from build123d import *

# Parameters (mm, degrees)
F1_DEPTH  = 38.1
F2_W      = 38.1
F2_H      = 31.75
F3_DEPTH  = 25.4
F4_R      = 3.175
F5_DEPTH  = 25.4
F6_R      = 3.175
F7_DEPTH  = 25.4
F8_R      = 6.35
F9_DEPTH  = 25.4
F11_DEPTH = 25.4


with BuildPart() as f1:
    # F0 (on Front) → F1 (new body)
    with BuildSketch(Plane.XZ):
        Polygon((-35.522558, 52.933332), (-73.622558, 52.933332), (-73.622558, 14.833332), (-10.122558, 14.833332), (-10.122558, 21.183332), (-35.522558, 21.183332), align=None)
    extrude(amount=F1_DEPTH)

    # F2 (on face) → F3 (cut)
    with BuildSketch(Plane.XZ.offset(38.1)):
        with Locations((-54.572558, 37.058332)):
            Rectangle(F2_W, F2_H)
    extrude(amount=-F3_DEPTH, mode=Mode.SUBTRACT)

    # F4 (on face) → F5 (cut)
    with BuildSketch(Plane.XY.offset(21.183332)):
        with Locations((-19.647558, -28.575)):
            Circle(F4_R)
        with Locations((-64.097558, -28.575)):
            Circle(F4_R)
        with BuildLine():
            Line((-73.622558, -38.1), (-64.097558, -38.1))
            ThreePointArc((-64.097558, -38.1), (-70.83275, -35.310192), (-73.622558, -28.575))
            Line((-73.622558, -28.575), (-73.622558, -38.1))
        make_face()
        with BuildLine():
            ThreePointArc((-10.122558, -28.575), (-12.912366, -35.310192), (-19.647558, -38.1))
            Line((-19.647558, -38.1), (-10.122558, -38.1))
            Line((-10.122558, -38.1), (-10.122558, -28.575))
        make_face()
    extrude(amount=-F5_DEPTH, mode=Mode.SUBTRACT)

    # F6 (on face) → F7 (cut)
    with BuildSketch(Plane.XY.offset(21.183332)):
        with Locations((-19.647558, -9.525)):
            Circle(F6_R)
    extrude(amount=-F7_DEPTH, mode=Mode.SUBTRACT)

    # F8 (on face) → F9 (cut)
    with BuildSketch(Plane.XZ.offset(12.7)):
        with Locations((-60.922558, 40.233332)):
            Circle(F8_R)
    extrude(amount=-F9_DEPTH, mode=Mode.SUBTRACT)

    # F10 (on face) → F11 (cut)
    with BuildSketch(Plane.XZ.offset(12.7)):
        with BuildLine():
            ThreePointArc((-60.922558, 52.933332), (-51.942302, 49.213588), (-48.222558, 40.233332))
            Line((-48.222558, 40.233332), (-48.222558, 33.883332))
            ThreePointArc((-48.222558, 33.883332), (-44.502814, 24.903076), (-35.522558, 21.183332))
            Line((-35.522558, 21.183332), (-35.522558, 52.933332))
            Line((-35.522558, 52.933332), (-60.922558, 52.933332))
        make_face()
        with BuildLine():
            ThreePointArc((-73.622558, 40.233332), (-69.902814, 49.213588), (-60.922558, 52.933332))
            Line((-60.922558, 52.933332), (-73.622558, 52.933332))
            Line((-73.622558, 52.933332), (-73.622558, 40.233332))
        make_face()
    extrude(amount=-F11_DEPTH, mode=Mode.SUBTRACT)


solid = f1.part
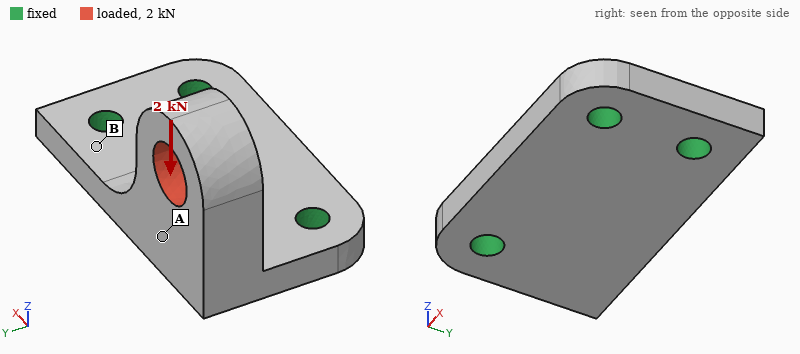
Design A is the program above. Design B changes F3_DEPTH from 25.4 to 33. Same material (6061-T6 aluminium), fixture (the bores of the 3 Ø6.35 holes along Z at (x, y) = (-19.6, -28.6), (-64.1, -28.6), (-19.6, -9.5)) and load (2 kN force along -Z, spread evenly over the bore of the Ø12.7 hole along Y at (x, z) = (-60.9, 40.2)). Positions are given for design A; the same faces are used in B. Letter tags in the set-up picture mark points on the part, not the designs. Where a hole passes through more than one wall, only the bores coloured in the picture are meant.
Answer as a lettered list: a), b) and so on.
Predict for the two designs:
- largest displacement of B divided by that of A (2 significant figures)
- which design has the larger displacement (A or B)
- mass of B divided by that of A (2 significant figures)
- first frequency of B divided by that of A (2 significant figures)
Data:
a) 1.7
b) B
c) 0.78
d) 1.0
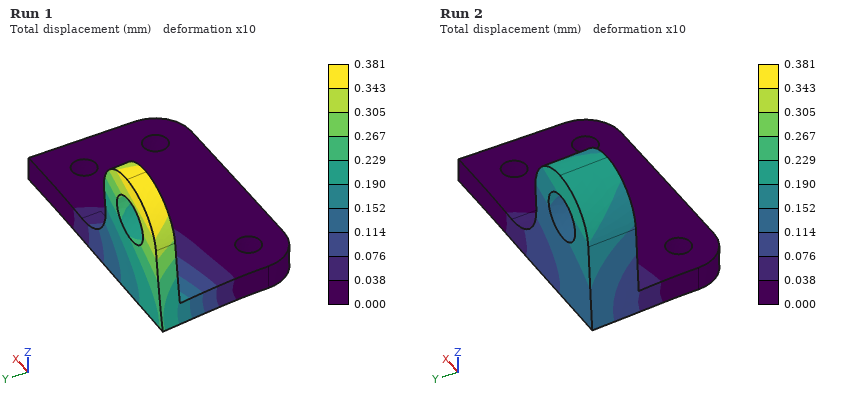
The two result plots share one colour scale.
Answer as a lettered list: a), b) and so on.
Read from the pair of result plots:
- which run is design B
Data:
a) Run 1
